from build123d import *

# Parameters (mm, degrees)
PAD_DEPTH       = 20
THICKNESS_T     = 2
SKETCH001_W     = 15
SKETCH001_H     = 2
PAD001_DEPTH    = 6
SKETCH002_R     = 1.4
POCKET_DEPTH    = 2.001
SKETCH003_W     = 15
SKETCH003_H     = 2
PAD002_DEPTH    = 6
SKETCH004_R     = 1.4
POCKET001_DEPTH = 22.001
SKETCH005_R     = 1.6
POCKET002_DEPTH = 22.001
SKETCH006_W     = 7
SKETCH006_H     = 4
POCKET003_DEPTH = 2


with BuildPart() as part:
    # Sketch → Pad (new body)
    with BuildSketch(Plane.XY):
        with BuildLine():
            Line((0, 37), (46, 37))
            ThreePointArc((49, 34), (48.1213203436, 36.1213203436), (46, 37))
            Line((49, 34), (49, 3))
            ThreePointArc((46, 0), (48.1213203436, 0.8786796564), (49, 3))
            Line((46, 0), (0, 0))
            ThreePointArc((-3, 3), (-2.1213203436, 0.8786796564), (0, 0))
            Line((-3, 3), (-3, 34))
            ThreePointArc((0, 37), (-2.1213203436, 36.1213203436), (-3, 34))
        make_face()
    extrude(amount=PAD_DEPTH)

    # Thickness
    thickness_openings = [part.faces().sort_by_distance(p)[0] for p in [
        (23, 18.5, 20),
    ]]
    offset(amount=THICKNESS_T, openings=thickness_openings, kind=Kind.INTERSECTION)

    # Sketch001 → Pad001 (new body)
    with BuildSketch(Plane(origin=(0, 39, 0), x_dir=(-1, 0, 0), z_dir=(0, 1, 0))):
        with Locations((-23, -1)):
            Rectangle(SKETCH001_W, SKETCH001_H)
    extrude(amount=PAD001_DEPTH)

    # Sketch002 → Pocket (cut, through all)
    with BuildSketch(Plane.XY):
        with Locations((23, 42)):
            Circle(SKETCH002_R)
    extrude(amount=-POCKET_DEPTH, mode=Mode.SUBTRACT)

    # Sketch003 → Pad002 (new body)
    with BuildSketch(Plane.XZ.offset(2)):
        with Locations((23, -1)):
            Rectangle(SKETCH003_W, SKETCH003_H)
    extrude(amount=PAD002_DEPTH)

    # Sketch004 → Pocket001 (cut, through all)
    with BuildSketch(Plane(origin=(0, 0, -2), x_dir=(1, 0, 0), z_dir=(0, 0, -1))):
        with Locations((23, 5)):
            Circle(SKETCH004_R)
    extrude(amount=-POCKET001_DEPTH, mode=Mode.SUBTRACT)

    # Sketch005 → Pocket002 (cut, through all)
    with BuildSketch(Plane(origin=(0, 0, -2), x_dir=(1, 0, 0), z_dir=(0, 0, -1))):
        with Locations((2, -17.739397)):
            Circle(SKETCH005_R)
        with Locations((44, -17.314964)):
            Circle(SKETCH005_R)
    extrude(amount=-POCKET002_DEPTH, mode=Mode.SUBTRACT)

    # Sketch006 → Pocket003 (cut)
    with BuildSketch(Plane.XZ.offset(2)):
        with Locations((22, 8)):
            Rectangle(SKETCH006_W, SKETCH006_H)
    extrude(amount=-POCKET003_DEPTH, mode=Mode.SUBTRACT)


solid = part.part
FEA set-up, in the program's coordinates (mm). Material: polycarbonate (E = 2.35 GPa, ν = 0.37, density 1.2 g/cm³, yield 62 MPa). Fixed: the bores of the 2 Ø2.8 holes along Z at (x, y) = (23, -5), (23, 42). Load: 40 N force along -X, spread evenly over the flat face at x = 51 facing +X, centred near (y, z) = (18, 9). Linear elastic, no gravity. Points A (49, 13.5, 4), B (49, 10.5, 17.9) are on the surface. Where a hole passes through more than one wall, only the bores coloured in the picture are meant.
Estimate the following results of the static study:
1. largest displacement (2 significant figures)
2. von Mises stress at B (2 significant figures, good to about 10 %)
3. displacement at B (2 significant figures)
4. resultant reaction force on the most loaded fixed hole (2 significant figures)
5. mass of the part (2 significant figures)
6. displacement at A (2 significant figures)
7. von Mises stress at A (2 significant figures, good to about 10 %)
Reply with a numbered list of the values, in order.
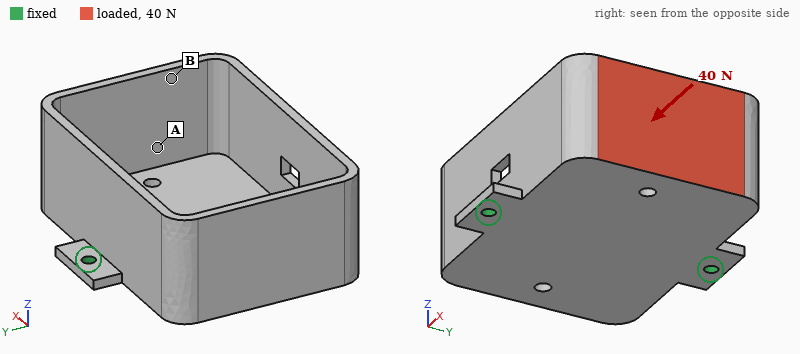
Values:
1. 0.84 mm
2. 4.1 MPa
3. 0.70 mm
4. 20 N
5. 14 g
6. 0.47 mm
7. 1.8 MPa
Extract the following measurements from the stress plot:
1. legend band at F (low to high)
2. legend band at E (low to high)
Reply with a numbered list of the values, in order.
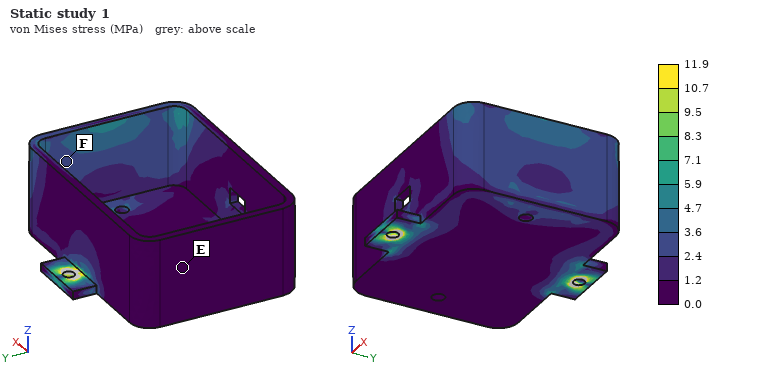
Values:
1. 2.4 to 3.6 MPa
2. 0.0 to 1.2 MPa
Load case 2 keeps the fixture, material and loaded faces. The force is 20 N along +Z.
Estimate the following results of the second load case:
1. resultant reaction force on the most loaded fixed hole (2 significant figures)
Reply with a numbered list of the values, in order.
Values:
1. 10 N
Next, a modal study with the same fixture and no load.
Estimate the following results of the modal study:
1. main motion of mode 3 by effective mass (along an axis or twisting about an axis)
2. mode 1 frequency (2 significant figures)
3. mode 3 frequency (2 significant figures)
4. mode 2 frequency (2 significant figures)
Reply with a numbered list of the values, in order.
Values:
1. along Z
2. 300 Hz
3. 1200 Hz
4. 670 Hz
